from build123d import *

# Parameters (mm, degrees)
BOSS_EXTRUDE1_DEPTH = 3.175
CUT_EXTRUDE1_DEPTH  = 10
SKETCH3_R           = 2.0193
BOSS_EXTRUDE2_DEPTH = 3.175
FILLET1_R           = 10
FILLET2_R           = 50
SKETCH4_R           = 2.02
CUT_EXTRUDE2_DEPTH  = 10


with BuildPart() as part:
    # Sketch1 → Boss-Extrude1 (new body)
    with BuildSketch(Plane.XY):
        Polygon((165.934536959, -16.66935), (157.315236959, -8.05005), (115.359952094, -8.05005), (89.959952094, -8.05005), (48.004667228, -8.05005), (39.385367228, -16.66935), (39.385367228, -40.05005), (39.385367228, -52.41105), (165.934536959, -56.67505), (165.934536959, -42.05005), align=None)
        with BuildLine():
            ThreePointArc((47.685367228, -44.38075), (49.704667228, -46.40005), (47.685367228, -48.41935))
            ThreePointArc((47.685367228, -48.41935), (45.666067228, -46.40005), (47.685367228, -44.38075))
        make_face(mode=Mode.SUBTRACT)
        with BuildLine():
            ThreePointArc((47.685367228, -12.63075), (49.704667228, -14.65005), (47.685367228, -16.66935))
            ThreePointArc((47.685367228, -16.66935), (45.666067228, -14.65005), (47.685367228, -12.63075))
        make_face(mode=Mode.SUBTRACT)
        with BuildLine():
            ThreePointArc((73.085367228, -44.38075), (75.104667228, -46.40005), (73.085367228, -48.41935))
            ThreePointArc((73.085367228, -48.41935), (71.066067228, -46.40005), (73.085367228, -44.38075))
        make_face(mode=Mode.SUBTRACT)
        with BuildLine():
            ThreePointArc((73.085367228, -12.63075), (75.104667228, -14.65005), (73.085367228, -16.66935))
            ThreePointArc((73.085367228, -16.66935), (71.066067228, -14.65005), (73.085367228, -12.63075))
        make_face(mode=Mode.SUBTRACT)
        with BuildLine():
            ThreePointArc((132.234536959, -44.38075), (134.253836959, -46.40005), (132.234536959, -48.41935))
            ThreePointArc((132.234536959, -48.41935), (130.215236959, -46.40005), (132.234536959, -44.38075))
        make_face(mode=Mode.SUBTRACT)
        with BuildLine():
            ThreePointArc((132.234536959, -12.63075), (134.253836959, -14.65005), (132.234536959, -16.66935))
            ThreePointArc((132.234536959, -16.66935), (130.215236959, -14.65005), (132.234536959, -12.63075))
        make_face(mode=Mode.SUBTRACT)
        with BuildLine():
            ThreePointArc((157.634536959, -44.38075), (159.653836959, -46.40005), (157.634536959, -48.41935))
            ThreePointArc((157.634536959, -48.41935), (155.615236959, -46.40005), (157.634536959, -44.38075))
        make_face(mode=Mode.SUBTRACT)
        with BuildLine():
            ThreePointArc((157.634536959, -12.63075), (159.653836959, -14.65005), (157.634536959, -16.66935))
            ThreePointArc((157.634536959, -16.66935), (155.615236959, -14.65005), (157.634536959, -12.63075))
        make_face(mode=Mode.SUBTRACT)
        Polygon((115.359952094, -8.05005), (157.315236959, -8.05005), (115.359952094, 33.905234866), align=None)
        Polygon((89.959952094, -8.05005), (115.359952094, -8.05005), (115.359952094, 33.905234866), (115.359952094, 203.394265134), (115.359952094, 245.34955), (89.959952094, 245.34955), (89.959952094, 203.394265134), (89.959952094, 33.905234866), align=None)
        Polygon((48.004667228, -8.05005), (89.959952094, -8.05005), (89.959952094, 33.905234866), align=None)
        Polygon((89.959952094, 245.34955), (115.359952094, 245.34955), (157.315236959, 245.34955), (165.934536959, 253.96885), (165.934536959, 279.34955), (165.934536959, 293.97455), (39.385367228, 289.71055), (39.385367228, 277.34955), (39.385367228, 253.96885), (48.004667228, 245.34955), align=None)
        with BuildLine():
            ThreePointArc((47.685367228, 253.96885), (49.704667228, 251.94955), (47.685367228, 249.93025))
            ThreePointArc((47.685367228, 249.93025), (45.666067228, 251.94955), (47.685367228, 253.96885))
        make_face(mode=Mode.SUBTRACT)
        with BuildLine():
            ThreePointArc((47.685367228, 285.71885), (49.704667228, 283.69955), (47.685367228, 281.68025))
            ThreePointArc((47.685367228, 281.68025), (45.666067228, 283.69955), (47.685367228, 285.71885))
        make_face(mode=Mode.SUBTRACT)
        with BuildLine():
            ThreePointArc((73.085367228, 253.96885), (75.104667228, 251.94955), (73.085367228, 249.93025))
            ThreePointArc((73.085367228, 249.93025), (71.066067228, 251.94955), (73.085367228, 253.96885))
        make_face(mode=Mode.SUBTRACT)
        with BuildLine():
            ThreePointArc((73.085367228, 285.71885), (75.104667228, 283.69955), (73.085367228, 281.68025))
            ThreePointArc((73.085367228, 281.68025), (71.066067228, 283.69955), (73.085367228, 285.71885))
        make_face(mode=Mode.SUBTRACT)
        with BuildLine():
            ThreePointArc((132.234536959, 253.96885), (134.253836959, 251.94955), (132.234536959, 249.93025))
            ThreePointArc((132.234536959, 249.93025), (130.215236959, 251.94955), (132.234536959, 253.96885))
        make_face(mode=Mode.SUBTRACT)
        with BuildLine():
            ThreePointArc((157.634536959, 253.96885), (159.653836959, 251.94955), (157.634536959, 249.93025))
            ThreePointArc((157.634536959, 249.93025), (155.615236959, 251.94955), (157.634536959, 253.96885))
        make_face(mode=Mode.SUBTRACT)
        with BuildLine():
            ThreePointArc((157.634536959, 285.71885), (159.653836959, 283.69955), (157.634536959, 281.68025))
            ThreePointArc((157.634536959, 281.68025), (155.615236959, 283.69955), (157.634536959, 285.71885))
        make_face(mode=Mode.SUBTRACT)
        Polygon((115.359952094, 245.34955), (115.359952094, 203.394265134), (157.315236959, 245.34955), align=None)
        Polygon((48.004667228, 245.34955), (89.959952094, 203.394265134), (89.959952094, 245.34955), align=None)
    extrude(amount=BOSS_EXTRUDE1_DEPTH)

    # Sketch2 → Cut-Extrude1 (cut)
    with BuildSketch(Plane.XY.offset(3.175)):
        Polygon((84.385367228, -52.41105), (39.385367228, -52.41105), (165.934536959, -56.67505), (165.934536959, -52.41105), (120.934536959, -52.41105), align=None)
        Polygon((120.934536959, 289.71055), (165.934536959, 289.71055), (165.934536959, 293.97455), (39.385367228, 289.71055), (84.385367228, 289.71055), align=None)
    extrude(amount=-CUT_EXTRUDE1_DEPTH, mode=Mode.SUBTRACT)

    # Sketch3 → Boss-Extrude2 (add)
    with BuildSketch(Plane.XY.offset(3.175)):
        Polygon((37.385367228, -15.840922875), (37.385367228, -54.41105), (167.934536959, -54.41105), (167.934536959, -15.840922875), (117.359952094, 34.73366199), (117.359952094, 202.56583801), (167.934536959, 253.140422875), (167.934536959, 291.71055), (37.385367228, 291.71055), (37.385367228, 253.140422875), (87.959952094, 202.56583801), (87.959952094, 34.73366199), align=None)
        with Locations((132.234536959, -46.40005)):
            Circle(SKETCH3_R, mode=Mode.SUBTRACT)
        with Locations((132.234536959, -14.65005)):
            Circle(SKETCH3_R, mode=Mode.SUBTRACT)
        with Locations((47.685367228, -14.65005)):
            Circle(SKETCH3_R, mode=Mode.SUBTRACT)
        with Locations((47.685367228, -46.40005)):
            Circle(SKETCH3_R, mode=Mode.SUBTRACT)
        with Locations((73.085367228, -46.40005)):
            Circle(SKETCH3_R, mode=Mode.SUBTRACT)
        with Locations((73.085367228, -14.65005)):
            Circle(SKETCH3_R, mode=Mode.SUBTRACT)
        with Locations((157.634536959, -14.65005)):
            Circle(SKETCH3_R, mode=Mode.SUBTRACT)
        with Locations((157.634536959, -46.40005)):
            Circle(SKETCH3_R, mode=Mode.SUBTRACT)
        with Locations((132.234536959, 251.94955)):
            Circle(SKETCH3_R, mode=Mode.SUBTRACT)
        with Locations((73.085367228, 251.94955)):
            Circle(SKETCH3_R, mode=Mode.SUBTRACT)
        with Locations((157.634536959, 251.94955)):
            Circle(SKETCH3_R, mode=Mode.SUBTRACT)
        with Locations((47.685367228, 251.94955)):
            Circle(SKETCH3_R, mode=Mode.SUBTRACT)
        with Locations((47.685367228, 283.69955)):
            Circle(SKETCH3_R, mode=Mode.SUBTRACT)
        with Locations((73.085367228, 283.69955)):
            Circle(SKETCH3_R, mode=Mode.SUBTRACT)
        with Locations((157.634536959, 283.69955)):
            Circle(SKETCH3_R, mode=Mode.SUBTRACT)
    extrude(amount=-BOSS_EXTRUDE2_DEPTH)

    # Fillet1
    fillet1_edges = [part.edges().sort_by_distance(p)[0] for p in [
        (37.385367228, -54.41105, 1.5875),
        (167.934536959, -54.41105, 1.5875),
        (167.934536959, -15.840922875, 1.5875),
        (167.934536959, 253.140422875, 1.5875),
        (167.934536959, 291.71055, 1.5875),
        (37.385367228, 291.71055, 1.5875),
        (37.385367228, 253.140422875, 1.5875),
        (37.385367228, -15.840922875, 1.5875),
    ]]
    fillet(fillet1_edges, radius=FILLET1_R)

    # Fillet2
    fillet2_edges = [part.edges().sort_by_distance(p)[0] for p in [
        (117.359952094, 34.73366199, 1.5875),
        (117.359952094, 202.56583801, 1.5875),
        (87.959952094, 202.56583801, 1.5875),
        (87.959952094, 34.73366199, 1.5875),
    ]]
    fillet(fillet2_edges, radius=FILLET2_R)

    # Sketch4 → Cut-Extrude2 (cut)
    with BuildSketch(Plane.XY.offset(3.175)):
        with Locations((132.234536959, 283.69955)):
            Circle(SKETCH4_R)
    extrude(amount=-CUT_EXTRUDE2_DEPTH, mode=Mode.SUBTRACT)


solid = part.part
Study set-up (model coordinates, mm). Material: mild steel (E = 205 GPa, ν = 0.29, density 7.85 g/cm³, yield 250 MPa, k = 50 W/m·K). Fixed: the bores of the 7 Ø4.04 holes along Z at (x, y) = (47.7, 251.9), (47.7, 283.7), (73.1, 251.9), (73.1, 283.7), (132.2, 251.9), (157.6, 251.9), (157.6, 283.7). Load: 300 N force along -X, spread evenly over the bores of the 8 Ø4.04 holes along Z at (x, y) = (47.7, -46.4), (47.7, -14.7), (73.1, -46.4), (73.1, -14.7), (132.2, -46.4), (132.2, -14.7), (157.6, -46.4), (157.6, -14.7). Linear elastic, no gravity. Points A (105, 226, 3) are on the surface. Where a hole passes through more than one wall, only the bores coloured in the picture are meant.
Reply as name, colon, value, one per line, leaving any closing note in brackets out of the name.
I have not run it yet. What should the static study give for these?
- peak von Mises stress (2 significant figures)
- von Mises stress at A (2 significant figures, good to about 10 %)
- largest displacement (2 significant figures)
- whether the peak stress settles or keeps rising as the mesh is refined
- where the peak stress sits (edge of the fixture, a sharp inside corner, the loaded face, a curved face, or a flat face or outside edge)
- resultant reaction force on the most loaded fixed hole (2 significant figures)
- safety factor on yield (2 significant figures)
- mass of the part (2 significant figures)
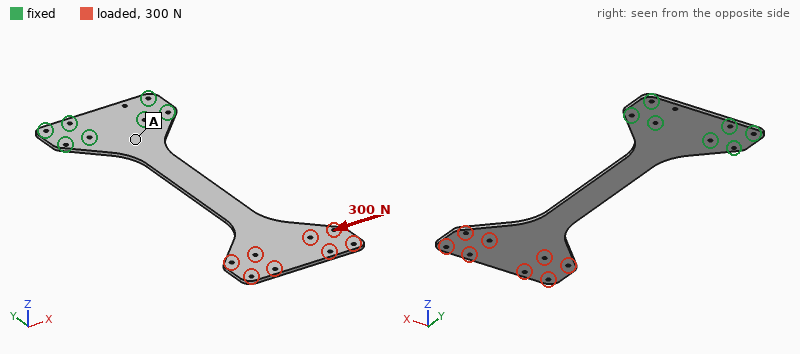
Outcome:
peak von Mises stress: 150 MPa
von Mises stress at A: 17 MPa
largest displacement: 1.2 mm
whether the peak stress settles or keeps rising as the mesh is refined: settles
where the peak stress sits: a curved face
resultant reaction force on the most loaded fixed hole: 760 N
safety factor on yield: 1.6
mass of the part: 570 g
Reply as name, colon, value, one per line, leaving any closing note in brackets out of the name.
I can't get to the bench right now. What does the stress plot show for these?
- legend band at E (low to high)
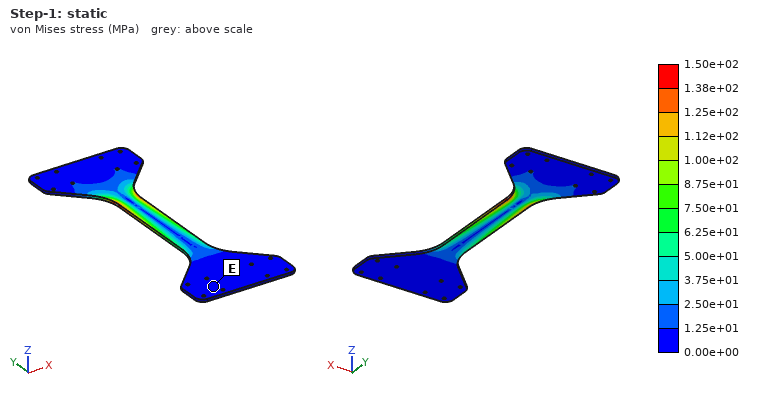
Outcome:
legend band at E: 0.00e+00 to 1.25e+01 MPa
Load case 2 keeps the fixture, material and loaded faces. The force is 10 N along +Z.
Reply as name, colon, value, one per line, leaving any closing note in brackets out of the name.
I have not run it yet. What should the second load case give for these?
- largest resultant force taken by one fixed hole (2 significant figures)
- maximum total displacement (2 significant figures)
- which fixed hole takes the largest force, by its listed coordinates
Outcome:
largest resultant force taken by one fixed hole: 32 N
maximum total displacement: 4.0 mm
which fixed hole takes the largest force, by its listed coordinates: (73.1, 251.9)
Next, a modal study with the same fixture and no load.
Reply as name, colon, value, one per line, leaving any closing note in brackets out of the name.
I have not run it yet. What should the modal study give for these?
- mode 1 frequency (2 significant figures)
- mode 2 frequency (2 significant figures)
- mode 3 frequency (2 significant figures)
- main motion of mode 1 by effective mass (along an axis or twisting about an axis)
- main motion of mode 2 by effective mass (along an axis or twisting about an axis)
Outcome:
mode 1 frequency: 19 Hz
mode 2 frequency: 110 Hz
mode 3 frequency: 170 Hz
main motion of mode 1 by effective mass: along Z
main motion of mode 2 by effective mass: twisting about Y
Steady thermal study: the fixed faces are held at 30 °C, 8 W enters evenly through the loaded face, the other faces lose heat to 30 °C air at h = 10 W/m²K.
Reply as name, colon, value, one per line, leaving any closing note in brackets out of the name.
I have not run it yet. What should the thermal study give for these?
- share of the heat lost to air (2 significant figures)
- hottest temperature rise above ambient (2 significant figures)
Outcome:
share of the heat lost to air: 97 %
hottest temperature rise above ambient: 42 K
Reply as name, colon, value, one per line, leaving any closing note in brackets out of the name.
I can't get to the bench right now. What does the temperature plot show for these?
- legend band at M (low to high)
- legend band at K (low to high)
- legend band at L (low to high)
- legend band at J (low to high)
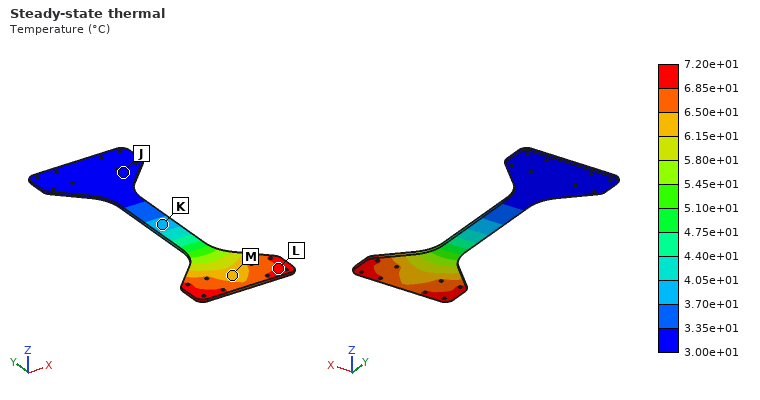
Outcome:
legend band at M: 6.15e+01 to 6.50e+01 °C
legend band at K: 3.70e+01 to 4.05e+01 °C
legend band at L: 6.85e+01 to 7.20e+01 °C
legend band at J: 3.00e+01 to 3.35e+01 °C
